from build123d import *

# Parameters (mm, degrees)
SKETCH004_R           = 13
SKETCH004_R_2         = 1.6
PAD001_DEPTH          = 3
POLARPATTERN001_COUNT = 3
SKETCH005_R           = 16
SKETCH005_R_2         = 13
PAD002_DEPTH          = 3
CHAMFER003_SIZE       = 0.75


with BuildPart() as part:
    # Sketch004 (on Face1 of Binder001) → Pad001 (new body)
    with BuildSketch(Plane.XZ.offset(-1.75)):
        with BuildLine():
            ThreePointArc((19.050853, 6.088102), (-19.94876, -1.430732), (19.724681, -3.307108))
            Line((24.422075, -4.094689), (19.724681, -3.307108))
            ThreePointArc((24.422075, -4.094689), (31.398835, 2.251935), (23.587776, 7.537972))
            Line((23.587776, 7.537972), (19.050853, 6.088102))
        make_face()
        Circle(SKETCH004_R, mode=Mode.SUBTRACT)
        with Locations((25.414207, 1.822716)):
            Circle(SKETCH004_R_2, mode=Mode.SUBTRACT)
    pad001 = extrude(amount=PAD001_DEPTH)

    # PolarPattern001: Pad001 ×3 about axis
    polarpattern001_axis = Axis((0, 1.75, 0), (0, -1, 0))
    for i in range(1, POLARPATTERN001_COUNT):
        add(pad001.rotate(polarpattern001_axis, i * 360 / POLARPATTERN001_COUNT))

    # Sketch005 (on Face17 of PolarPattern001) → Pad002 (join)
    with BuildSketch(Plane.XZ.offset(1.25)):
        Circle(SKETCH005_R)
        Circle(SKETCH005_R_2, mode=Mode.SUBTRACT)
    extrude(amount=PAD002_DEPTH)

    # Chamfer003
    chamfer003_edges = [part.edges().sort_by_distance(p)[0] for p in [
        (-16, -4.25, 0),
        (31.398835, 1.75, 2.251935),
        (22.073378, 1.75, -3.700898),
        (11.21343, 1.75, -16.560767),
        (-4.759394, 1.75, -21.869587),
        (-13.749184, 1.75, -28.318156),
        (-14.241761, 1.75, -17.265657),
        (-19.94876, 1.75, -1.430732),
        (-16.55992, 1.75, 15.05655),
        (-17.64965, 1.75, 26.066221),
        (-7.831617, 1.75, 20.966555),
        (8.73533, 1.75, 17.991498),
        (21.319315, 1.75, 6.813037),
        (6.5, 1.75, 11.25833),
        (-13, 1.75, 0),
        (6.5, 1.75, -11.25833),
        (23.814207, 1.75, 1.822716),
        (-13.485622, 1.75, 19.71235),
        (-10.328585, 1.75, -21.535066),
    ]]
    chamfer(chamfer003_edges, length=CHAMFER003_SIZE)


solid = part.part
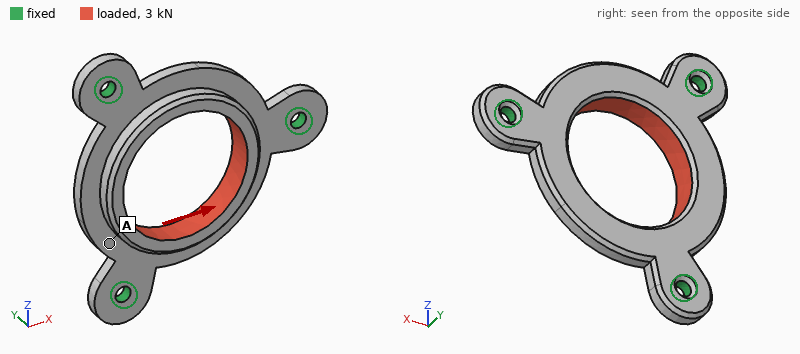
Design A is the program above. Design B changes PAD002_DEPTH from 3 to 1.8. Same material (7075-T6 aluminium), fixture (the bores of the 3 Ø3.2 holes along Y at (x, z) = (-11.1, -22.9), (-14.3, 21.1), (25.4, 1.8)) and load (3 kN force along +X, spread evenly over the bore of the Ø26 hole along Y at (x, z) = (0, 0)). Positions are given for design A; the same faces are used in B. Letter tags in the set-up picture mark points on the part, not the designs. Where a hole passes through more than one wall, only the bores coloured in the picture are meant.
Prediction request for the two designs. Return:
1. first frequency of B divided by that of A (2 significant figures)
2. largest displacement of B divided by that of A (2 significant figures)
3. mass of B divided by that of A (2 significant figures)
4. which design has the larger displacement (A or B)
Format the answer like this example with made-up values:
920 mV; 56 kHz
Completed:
0.97; 0.92; 0.92; A
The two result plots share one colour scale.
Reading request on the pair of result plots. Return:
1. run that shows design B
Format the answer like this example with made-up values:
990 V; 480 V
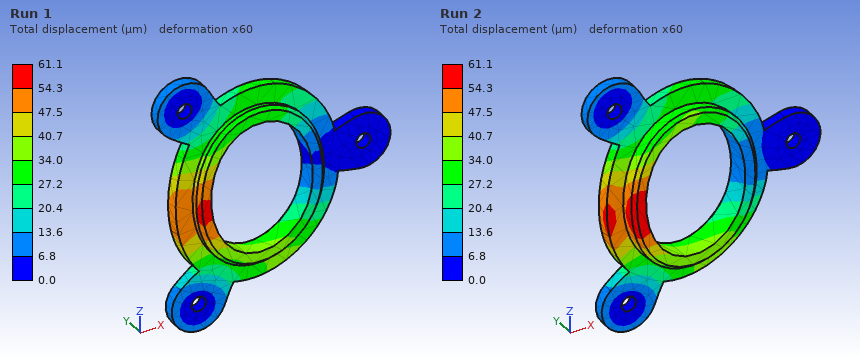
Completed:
Run 1
